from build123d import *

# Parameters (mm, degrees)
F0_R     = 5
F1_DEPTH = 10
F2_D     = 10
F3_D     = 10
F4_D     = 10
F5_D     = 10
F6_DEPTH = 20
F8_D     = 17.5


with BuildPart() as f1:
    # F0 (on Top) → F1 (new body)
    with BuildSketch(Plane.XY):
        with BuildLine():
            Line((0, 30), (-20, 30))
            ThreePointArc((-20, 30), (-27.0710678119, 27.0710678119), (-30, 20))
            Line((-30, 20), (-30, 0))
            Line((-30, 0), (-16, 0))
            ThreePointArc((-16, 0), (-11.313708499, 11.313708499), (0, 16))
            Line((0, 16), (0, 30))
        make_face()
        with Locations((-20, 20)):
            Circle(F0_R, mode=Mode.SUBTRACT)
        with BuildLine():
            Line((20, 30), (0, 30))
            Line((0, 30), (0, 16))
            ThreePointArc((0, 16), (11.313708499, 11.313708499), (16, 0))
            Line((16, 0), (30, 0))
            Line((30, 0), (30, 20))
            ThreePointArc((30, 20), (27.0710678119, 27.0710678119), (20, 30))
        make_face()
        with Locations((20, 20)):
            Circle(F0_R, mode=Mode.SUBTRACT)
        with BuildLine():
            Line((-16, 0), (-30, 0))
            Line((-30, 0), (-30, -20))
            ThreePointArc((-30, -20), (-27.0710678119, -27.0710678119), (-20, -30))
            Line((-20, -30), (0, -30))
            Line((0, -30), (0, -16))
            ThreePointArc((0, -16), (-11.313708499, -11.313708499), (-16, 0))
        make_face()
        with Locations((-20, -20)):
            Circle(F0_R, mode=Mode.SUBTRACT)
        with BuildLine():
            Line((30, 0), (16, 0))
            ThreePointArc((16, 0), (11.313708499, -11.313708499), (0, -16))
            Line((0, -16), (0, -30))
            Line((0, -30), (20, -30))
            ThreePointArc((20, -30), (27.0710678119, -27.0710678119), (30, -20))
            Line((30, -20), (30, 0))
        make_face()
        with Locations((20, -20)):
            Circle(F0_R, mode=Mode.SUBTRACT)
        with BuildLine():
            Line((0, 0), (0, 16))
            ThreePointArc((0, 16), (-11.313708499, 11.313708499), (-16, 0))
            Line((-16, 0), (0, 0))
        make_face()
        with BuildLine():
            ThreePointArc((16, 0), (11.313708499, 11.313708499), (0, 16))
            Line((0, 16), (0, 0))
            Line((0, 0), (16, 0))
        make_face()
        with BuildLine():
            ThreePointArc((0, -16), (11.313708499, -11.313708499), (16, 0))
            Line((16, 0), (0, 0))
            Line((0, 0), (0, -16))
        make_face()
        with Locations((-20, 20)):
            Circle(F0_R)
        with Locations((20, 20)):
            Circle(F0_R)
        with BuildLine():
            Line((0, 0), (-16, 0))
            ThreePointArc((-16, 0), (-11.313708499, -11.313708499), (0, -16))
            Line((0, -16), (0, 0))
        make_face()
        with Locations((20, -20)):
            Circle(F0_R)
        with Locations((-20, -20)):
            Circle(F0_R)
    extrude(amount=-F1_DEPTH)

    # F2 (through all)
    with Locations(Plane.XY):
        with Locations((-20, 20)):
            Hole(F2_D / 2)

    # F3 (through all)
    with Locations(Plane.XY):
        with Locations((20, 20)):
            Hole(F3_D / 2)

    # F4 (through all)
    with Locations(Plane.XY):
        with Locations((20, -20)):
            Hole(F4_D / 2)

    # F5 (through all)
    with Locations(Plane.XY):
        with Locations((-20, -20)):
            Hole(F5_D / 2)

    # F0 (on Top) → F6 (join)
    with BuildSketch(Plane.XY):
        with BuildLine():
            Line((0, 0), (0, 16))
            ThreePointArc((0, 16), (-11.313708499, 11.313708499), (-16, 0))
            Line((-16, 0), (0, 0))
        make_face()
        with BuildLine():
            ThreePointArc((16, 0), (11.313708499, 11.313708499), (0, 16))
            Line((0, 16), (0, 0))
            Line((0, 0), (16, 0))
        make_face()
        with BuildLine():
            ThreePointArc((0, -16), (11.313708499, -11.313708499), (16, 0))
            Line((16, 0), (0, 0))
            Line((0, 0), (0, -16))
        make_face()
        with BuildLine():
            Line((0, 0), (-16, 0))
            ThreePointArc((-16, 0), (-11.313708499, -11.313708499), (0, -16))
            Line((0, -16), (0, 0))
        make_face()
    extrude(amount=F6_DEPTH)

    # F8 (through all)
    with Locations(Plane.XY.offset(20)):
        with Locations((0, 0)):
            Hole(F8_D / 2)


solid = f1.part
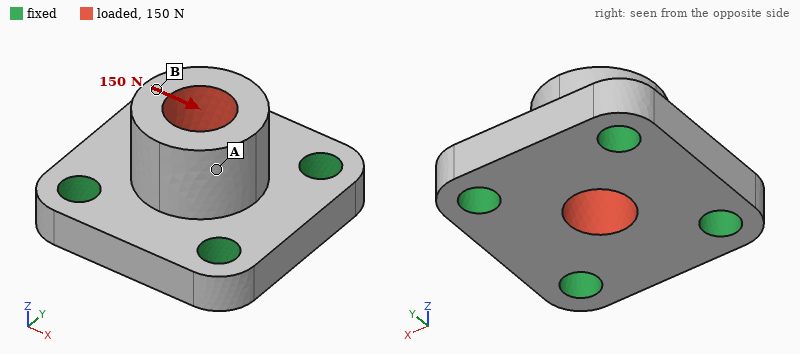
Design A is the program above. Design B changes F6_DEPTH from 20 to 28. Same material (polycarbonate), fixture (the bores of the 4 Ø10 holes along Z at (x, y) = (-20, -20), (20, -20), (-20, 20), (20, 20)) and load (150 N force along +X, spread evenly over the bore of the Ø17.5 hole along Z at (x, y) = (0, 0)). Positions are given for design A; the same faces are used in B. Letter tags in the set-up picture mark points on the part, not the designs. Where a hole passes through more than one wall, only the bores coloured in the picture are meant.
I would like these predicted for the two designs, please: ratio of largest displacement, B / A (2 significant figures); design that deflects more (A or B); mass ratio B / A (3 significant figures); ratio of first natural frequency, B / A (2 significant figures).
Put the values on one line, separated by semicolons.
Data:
1.7; B; 1.11; 0.69
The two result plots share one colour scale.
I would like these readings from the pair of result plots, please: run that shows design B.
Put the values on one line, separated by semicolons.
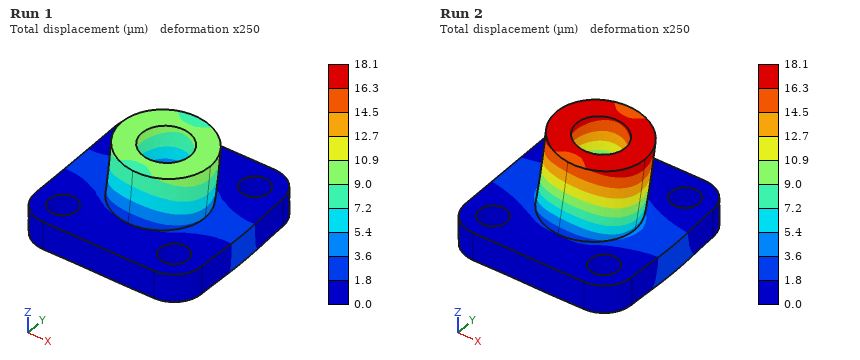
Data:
Run 2
